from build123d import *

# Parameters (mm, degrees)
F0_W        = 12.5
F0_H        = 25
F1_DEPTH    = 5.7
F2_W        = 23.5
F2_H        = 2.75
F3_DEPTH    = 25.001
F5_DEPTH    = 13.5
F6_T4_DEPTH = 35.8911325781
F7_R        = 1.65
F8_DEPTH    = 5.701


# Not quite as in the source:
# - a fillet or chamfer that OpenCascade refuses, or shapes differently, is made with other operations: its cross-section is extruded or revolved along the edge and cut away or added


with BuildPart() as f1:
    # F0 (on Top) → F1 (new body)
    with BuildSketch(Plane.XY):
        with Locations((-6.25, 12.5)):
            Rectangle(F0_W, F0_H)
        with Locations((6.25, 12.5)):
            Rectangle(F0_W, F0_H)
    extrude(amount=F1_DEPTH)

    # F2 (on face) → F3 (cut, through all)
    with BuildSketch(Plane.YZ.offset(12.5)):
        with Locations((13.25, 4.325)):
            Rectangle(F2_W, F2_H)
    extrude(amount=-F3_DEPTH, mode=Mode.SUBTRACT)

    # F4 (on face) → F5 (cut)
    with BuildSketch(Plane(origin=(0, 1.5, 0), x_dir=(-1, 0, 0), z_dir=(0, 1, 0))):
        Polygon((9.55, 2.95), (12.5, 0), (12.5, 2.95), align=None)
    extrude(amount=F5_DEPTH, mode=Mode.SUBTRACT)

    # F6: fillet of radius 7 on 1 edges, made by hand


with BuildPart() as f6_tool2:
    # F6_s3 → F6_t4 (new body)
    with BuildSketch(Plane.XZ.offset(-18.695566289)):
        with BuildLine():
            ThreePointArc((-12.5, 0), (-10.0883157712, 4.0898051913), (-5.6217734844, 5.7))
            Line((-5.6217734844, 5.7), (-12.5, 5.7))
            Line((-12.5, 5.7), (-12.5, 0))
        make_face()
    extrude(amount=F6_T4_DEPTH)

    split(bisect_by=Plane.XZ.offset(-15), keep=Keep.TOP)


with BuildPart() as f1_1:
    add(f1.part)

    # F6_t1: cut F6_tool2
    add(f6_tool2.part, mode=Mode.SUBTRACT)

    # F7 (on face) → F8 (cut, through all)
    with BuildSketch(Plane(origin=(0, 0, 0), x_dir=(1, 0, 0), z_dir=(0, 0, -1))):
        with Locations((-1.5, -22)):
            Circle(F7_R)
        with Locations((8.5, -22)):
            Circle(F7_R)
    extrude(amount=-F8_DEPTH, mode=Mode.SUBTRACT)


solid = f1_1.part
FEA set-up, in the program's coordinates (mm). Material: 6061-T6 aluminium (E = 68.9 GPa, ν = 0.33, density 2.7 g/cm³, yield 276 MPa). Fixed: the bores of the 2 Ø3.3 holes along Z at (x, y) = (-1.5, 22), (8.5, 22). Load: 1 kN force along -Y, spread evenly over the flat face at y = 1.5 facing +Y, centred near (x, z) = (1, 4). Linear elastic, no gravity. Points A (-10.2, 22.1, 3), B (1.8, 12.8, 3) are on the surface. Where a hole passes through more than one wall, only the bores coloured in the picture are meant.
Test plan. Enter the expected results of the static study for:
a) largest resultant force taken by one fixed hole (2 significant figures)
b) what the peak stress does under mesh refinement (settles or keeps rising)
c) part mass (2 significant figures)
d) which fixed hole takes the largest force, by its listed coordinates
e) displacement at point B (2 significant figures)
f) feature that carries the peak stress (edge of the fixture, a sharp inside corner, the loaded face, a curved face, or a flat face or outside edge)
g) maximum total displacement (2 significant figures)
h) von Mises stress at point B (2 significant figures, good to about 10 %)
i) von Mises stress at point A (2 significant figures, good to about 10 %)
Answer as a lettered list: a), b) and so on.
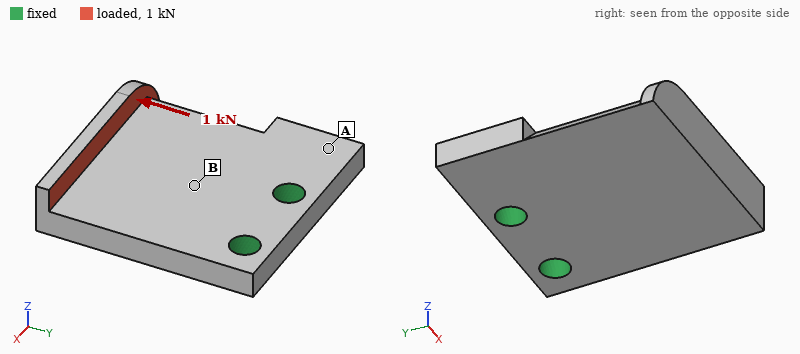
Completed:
a) 700 N
b) keeps rising
c) 4.9 g
d) (-1.5, 22)
e) 0.034 mm
f) edge of the fixture
g) 0.20 mm
h) 91 MPa
i) 19 MPa
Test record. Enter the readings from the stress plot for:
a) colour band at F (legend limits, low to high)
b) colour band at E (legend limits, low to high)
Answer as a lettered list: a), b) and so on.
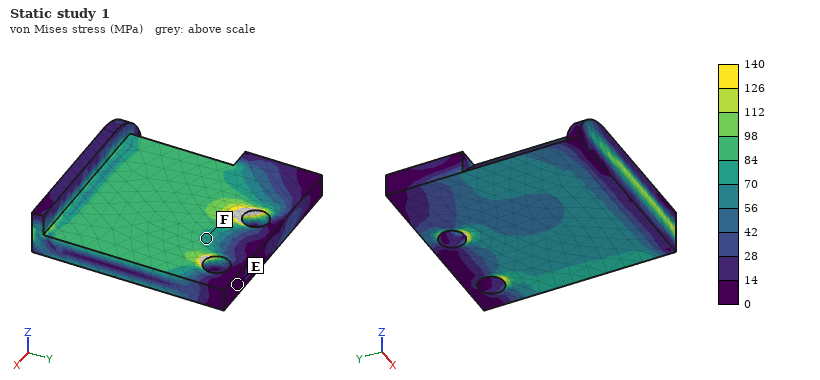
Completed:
a) 70 to 84 MPa
b) 0 to 14 MPa
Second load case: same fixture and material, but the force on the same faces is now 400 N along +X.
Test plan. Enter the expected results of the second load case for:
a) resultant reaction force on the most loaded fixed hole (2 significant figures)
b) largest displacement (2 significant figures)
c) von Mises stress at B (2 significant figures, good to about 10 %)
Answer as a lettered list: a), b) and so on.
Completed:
a) 670 N
b) 57 µm
c) 46 MPa
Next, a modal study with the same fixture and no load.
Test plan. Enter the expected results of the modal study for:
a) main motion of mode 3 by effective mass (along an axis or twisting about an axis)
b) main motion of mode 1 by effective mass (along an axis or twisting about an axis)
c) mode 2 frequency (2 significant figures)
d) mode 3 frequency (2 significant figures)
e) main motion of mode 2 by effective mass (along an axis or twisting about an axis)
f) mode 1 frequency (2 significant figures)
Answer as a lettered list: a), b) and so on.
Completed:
a) along X
b) along Z
c) 9500 Hz
d) 17 kHz
e) twisting about Y
f) 4600 Hz
